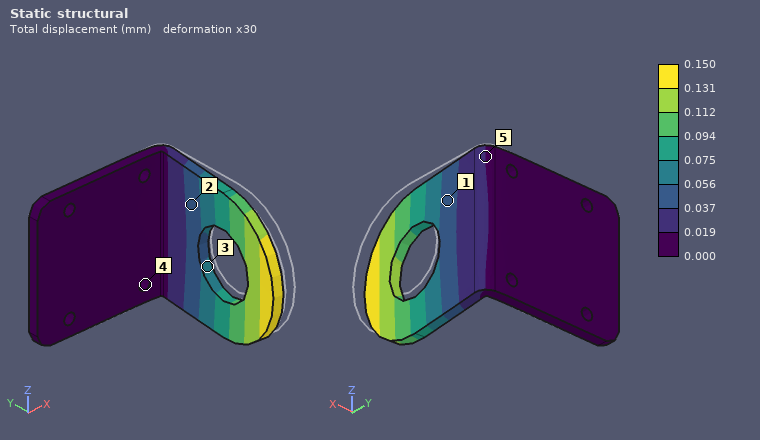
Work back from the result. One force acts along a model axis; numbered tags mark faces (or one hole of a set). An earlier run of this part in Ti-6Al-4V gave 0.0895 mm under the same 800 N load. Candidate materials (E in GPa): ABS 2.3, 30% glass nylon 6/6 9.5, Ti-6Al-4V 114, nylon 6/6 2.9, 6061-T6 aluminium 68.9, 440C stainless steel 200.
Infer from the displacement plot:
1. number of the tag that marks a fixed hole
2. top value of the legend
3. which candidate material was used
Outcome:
4
0.150 mm
6061-T6 aluminium
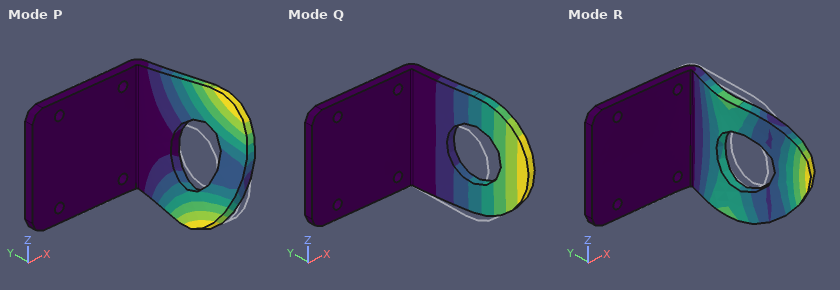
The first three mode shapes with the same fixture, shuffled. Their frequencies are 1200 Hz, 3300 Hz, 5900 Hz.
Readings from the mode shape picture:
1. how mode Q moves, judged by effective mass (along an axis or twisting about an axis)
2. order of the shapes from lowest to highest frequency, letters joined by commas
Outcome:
along X
Q, P, R
